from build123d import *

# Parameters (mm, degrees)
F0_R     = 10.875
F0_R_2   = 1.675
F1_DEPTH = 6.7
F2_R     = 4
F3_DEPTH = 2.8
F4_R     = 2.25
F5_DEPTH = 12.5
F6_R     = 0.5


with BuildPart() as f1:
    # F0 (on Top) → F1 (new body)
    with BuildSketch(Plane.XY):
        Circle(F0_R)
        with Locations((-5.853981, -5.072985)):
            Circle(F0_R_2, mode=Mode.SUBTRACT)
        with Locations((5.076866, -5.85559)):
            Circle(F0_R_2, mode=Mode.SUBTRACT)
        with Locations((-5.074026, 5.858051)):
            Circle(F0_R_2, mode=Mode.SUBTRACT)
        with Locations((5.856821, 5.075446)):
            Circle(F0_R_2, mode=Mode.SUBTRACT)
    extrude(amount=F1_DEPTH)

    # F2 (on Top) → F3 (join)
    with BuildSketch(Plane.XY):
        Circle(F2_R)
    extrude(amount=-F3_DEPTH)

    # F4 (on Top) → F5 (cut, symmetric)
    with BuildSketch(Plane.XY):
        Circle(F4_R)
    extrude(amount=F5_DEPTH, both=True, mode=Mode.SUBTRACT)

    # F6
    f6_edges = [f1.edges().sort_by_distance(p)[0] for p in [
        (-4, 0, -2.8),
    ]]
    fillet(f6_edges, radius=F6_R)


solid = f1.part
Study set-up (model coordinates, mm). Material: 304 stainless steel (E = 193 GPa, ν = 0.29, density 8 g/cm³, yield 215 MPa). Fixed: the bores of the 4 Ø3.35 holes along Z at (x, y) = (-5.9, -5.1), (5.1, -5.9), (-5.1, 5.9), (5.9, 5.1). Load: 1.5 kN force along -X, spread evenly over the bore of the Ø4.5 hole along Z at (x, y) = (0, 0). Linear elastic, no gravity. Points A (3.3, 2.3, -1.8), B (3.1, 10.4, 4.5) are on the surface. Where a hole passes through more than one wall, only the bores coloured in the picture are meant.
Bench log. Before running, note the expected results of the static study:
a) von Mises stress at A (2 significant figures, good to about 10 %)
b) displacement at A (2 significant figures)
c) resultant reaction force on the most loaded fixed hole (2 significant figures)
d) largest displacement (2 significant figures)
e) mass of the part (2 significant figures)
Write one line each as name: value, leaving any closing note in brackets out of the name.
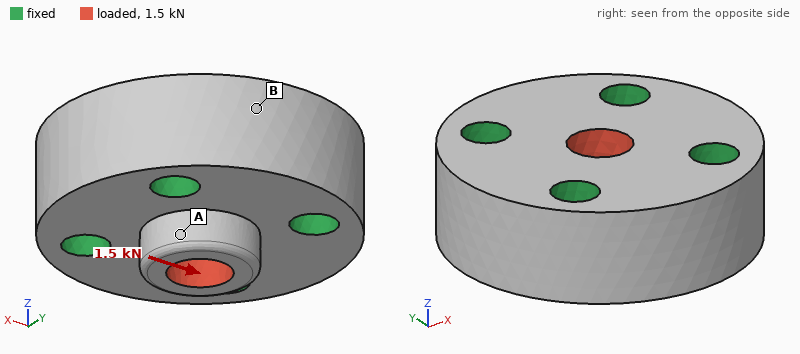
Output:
von Mises stress at A: 10 MPa
displacement at A: 0.87 µm
resultant reaction force on the most loaded fixed hole: 420 N
largest displacement: 1.3 µm
mass of the part: 18 g
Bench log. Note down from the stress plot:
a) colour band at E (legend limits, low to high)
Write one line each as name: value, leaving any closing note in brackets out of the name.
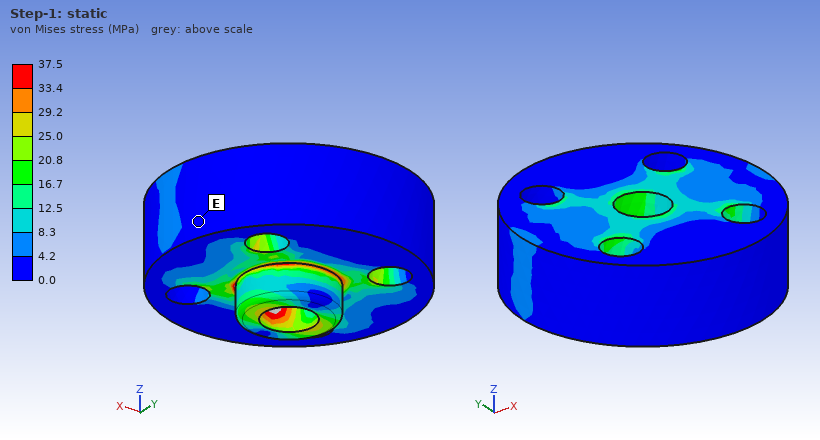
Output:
colour band at E: 0.0 to 4.2 MPa
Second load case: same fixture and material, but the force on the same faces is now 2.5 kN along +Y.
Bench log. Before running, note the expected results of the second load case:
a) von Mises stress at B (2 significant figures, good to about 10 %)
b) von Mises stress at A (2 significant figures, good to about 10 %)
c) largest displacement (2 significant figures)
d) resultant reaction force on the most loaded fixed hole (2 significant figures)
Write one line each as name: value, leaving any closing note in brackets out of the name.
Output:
von Mises stress at B: 5.9 MPa
von Mises stress at A: 13 MPa
largest displacement: 2.1 µm
resultant reaction force on the most loaded fixed hole: 710 N
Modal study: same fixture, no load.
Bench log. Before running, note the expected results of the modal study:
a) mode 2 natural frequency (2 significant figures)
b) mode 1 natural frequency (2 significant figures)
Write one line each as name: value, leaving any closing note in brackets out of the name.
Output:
mode 2 natural frequency: 110 kHz
mode 1 natural frequency: 110 kHz
